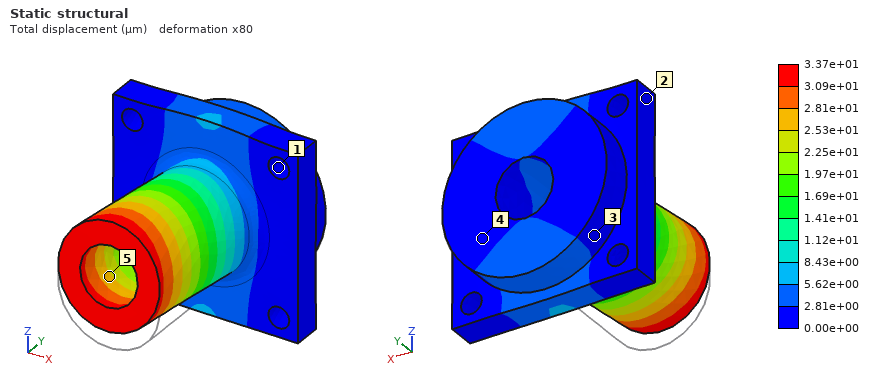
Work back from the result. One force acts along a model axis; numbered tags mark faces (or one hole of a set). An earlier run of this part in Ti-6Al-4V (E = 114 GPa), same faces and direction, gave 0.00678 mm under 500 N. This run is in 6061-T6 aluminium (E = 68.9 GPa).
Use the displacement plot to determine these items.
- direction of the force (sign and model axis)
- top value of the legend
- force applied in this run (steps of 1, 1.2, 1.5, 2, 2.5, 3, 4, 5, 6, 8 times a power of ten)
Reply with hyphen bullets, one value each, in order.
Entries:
- +Z
- 3.37e+01 µm
- 1.5 kN
